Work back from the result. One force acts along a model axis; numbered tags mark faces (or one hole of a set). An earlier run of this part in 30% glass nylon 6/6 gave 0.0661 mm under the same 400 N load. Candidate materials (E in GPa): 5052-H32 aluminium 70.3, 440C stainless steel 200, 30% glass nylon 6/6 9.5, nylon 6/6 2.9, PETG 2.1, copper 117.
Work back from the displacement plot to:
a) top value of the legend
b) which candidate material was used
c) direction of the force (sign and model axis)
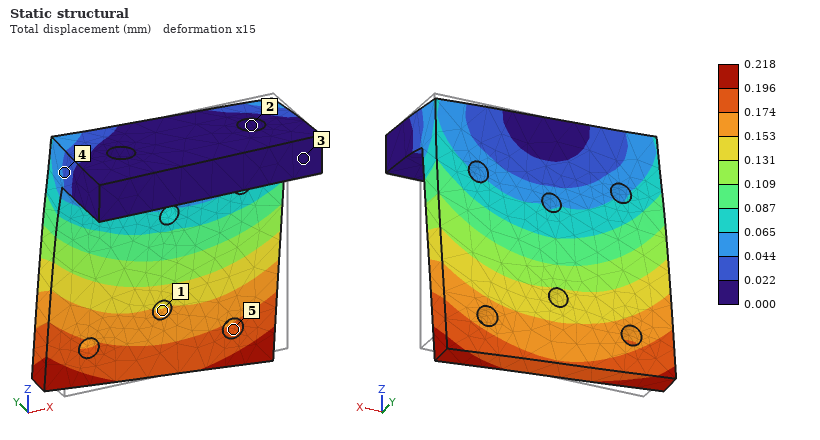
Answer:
0.218 mm
nylon 6/6
-X
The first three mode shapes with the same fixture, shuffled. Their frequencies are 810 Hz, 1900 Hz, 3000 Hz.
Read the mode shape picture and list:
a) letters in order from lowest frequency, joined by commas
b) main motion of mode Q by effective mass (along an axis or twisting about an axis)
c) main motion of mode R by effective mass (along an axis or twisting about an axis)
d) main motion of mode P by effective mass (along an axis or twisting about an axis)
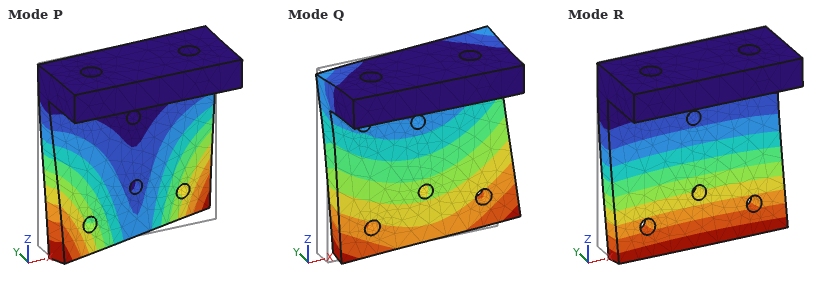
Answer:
R, P, Q
along X
along Y
twisting about Z
